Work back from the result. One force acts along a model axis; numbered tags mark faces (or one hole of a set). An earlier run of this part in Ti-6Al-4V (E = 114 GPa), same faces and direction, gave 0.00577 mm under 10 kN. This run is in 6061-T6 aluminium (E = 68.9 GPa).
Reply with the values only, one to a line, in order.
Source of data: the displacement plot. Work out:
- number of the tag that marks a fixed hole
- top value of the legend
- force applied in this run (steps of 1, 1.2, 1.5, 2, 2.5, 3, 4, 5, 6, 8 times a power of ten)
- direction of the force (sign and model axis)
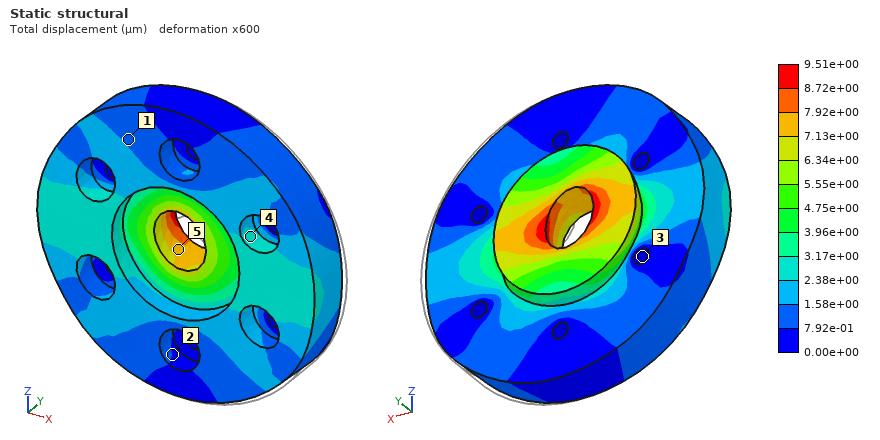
3
9.51e+00 µm
10 kN
-X
